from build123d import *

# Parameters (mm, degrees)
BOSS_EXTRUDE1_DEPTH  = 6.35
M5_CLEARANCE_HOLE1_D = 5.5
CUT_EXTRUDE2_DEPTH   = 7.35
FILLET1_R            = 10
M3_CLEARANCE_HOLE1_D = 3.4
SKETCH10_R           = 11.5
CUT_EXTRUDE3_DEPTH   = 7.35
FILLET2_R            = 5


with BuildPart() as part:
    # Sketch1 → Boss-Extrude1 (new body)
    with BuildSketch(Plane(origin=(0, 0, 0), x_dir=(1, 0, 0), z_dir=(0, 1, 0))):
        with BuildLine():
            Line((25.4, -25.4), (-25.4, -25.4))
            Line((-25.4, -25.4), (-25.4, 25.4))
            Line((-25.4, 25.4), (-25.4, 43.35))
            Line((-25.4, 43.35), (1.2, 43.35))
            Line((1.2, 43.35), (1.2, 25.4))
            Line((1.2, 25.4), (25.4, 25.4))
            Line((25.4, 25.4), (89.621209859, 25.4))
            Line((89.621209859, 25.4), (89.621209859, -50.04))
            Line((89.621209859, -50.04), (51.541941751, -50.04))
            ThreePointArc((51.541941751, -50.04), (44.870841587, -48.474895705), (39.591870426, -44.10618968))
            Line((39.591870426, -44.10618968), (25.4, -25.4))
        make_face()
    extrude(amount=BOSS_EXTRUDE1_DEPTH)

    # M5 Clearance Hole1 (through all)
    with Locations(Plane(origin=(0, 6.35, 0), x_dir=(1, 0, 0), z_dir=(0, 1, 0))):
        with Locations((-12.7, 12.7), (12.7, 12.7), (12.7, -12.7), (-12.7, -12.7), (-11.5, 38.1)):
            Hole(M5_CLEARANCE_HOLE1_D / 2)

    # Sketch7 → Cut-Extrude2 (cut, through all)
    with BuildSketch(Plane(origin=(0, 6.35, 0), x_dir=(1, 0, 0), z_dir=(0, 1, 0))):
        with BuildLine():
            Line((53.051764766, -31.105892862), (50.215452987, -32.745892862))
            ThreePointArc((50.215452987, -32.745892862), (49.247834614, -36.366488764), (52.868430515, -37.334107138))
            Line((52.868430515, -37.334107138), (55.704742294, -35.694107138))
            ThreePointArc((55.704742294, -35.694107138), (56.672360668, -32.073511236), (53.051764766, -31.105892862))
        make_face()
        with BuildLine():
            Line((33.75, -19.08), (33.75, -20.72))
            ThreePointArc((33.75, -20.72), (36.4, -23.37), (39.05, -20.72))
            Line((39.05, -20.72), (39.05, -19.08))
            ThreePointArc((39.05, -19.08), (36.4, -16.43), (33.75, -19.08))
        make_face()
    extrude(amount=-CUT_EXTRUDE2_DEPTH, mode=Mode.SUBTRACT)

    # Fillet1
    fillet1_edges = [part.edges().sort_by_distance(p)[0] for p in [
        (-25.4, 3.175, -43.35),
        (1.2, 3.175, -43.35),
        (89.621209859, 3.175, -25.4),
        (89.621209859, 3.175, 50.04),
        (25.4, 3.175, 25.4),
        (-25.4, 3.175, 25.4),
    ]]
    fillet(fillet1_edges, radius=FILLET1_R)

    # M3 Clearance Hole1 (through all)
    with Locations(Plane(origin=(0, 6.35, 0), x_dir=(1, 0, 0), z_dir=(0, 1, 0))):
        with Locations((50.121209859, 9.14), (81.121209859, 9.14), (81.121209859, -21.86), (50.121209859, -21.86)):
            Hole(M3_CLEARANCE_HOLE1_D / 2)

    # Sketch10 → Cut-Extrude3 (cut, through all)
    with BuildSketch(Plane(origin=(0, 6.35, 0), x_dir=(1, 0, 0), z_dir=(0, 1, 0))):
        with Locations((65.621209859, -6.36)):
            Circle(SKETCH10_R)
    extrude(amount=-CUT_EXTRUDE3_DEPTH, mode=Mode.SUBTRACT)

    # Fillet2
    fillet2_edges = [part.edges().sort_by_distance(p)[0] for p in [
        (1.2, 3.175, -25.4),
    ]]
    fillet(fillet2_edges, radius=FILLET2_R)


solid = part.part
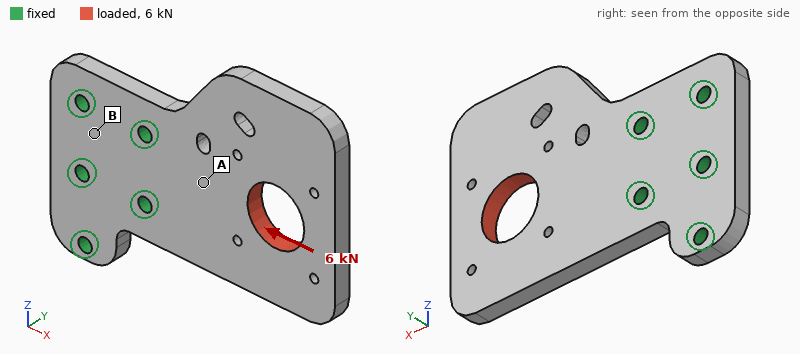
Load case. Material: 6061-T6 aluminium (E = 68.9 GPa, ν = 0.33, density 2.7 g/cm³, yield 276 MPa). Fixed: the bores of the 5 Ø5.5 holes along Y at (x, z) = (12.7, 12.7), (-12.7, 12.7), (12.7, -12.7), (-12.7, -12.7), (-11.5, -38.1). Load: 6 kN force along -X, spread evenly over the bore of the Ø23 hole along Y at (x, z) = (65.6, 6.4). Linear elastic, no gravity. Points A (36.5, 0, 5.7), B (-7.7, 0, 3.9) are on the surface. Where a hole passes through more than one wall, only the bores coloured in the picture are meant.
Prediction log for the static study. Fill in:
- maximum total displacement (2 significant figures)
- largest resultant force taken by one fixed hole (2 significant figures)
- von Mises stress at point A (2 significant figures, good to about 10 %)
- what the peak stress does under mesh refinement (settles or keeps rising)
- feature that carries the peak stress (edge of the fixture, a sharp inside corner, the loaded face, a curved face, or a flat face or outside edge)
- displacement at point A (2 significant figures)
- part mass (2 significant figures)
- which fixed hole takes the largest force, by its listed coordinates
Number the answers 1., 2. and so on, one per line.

1. 36 µm
2. 3.5 kN
3. 20 MPa
4. keeps rising
5. edge of the fixture
6. 8.8 µm
7. 120 g
8. (12.7, 12.7)
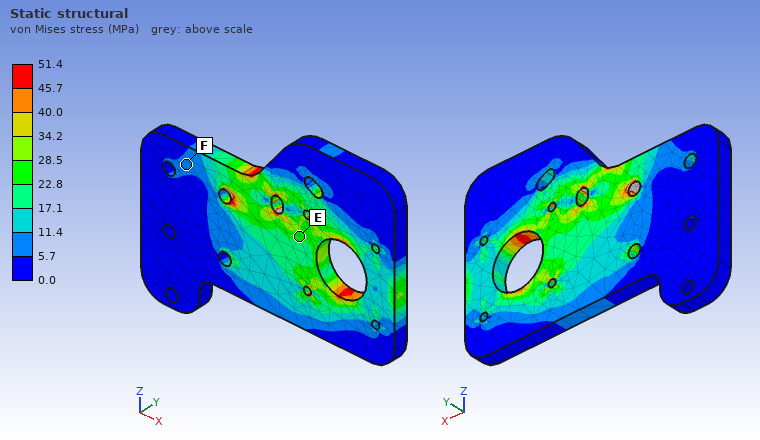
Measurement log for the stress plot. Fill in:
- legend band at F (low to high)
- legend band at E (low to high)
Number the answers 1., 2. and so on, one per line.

1. 5.7 to 11.4 MPa
2. 22.8 to 28.5 MPa
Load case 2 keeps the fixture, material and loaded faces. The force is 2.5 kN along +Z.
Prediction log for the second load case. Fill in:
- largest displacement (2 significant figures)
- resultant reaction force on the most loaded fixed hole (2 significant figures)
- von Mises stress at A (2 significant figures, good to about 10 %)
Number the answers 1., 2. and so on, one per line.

1. 93 µm
2. 3.6 kN
3. 27 MPa
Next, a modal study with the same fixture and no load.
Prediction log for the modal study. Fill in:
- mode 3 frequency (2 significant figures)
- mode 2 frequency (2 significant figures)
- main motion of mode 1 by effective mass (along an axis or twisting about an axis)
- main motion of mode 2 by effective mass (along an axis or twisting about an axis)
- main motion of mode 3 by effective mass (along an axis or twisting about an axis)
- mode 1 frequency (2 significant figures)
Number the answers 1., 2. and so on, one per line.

1. 3900 Hz
2. 1700 Hz
3. along Y
4. twisting about X
5. along Z
6. 770 Hz
